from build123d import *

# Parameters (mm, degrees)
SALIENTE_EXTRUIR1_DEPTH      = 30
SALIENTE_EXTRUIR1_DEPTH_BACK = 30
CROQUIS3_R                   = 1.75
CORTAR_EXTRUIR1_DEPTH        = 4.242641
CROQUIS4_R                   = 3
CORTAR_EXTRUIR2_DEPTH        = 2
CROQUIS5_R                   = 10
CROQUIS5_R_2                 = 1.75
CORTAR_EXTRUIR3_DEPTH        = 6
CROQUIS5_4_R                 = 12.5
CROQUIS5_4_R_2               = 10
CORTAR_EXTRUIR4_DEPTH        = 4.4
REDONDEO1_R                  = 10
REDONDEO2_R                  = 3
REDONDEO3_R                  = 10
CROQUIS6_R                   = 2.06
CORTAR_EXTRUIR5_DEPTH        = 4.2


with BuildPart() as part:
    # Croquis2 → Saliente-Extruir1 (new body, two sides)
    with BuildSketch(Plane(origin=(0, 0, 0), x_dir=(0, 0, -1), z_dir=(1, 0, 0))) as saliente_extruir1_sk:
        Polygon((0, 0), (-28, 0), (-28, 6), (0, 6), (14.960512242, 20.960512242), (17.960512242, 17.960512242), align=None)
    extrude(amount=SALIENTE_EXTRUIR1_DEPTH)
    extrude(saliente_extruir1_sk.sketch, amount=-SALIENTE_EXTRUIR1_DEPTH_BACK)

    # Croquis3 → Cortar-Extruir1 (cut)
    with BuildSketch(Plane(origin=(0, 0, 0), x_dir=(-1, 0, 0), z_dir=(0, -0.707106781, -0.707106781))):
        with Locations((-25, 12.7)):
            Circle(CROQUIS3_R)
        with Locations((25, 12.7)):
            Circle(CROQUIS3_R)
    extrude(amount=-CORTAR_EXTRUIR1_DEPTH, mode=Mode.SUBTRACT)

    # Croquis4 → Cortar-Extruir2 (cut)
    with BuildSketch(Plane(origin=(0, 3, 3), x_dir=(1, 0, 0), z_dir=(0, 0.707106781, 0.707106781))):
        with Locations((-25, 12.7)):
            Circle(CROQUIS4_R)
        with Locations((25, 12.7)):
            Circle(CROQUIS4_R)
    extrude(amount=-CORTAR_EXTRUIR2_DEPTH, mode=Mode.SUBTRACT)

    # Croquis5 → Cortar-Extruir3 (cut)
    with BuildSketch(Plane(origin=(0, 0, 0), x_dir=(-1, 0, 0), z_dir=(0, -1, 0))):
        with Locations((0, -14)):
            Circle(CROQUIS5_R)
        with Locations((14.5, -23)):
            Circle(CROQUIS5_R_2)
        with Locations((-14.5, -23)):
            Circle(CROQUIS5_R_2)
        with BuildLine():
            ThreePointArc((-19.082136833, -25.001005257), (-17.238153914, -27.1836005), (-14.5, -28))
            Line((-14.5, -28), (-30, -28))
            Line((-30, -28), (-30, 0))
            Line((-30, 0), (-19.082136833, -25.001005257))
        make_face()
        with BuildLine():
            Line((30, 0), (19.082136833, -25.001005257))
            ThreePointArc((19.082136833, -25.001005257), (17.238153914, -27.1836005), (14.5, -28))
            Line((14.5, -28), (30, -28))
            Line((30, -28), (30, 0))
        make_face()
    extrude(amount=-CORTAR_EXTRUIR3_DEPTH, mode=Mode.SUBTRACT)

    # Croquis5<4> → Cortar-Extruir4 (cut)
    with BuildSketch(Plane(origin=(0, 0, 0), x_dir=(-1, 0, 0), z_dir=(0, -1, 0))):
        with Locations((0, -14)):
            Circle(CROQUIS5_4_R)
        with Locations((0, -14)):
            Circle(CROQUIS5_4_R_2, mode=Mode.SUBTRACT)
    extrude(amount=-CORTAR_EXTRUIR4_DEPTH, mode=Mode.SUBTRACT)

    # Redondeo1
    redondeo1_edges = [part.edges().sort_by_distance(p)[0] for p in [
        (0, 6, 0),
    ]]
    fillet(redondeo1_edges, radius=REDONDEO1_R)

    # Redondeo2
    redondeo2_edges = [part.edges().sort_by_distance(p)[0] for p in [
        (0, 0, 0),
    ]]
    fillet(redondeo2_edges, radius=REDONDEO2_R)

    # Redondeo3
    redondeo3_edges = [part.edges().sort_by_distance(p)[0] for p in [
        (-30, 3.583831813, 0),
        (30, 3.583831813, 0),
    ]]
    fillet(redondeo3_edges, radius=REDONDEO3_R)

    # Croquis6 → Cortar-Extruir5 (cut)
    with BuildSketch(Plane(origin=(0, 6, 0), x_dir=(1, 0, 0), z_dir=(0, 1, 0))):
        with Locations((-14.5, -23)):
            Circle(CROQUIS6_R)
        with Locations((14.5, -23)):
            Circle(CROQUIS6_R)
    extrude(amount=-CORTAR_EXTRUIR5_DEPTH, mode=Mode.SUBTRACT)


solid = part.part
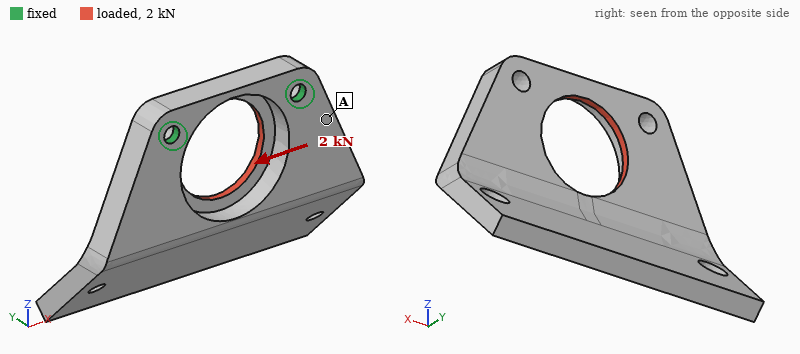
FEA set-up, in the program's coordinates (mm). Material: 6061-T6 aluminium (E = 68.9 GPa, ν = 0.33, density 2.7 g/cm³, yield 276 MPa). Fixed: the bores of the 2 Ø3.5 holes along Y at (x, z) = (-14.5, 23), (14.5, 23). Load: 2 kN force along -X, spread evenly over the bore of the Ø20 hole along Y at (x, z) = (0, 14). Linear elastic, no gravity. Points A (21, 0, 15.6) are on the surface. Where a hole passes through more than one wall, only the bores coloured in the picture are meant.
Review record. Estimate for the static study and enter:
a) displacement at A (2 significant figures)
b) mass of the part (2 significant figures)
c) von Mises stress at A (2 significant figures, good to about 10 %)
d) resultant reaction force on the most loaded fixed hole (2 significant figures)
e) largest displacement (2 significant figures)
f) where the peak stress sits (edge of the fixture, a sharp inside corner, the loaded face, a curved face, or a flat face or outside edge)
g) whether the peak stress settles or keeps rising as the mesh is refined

17 µm
30 g
19 MPa
1.1 kN
49 µm
edge of the fixture
keeps rising
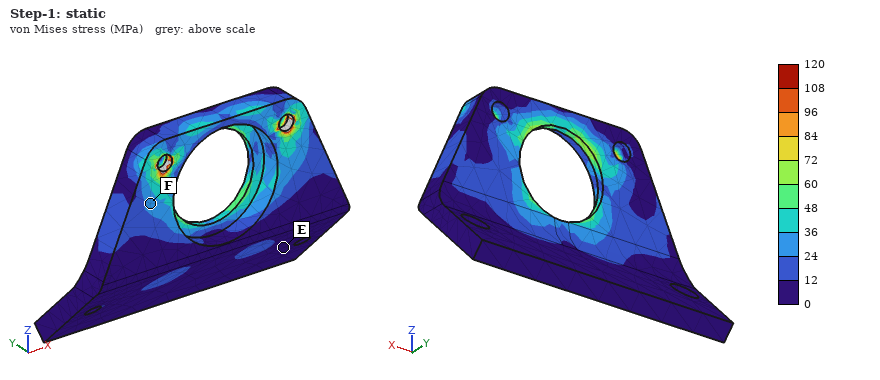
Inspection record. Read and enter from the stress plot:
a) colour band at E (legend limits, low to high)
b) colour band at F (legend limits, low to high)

0 to 12 MPa
24 to 36 MPa
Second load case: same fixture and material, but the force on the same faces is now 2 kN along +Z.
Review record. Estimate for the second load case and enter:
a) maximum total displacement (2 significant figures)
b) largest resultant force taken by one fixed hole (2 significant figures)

0.23 mm
1.0 kN
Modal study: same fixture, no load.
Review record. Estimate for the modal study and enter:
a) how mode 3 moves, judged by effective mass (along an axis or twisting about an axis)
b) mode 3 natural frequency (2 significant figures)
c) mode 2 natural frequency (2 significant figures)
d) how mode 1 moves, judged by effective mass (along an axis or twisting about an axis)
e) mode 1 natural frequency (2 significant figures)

along X
4900 Hz
2700 Hz
along Y
1300 Hz
